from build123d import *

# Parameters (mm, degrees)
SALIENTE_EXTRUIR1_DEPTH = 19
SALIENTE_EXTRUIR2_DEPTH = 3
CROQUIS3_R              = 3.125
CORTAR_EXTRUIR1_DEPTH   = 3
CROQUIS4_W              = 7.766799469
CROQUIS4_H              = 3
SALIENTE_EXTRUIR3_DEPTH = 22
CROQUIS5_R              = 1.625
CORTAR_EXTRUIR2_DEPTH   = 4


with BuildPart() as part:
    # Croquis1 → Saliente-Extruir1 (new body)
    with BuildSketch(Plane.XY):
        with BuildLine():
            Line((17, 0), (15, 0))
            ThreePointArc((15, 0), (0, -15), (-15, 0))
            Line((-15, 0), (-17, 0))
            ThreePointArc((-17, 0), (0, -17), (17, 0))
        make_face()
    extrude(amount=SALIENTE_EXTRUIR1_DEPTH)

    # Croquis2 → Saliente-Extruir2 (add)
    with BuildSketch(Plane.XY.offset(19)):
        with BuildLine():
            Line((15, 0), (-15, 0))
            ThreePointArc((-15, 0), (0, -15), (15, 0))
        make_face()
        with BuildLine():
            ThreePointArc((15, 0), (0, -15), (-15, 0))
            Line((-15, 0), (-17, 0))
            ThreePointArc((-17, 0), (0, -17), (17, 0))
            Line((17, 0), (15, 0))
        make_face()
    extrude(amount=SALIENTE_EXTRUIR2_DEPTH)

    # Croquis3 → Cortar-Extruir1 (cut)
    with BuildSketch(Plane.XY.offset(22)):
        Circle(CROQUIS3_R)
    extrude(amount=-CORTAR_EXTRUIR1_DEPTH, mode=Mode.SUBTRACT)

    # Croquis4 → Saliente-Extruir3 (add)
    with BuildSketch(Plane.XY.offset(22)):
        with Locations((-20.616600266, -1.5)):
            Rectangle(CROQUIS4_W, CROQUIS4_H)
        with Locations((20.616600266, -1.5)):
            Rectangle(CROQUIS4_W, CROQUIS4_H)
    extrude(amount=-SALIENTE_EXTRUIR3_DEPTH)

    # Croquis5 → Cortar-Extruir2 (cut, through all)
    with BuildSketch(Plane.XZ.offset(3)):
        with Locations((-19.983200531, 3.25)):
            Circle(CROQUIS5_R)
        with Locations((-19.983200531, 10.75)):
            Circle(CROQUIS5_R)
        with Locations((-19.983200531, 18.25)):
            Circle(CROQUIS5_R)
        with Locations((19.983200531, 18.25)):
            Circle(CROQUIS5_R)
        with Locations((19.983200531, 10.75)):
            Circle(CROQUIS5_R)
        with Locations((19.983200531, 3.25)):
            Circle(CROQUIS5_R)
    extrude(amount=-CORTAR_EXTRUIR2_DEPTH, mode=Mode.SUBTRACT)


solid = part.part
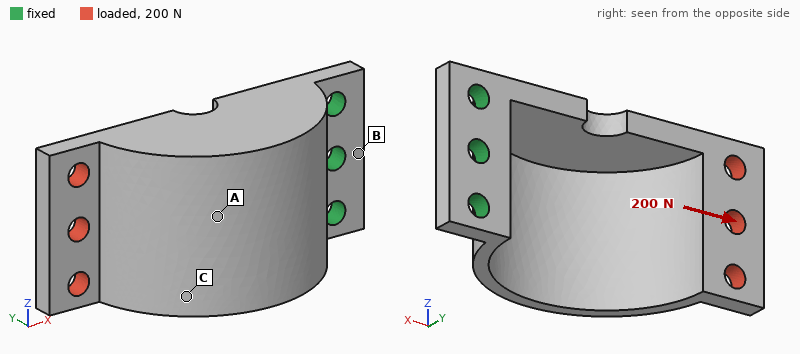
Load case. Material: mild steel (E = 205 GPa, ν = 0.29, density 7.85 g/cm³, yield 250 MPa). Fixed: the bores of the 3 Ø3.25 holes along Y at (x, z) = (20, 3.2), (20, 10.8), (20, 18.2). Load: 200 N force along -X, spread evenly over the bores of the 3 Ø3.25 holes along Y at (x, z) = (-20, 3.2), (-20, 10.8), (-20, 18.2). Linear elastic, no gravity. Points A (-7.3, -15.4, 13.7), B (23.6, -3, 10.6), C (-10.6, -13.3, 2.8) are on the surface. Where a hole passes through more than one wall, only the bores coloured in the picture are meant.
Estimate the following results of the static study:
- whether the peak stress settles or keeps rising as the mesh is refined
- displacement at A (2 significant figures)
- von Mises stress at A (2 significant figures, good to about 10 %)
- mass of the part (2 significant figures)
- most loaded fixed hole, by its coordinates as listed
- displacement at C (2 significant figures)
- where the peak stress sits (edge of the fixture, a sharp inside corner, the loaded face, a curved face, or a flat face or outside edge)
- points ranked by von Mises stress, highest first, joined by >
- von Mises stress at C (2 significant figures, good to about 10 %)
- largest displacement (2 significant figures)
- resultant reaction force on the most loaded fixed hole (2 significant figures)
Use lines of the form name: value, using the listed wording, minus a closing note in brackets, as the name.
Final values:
whether the peak stress settles or keeps rising as the mesh is refined: keeps rising
displacement at A: 0.030 mm
von Mises stress at A: 24 MPa
mass of the part: 32 g
most loaded fixed hole, by its coordinates as listed: (20, 18.2)
displacement at C: 0.040 mm
where the peak stress sits: a sharp inside corner
points ranked by von Mises stress, highest first, joined by >: C > A > B
von Mises stress at C: 39 MPa
largest displacement: 0.12 mm
resultant reaction force on the most loaded fixed hole: 87 N
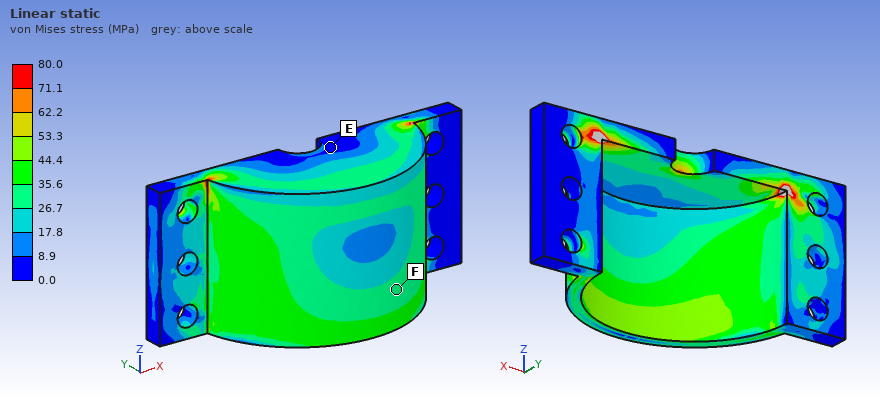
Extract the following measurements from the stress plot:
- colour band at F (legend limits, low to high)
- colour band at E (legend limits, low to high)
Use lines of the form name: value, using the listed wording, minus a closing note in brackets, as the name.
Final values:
colour band at F: 26.7 to 35.6 MPa
colour band at E: 0.0 to 8.9 MPa
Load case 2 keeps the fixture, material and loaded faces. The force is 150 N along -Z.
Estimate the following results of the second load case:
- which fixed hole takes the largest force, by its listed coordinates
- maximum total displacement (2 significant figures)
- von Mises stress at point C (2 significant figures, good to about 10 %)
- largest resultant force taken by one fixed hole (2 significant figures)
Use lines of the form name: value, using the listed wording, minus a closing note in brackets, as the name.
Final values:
which fixed hole takes the largest force, by its listed coordinates: (20, 18.2)
maximum total displacement: 0.23 mm
von Mises stress at point C: 31 MPa
largest resultant force taken by one fixed hole: 400 N
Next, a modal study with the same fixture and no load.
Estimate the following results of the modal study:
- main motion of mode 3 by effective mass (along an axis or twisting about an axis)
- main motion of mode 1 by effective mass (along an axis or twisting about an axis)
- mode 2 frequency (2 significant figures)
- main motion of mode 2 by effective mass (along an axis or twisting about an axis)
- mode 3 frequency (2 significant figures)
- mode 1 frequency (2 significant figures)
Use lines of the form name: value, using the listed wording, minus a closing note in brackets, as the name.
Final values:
main motion of mode 3 by effective mass: along X
main motion of mode 1 by effective mass: along Y
mode 2 frequency: 1600 Hz
main motion of mode 2 by effective mass: along Z
mode 3 frequency: 4400 Hz
mode 1 frequency: 1100 Hz
